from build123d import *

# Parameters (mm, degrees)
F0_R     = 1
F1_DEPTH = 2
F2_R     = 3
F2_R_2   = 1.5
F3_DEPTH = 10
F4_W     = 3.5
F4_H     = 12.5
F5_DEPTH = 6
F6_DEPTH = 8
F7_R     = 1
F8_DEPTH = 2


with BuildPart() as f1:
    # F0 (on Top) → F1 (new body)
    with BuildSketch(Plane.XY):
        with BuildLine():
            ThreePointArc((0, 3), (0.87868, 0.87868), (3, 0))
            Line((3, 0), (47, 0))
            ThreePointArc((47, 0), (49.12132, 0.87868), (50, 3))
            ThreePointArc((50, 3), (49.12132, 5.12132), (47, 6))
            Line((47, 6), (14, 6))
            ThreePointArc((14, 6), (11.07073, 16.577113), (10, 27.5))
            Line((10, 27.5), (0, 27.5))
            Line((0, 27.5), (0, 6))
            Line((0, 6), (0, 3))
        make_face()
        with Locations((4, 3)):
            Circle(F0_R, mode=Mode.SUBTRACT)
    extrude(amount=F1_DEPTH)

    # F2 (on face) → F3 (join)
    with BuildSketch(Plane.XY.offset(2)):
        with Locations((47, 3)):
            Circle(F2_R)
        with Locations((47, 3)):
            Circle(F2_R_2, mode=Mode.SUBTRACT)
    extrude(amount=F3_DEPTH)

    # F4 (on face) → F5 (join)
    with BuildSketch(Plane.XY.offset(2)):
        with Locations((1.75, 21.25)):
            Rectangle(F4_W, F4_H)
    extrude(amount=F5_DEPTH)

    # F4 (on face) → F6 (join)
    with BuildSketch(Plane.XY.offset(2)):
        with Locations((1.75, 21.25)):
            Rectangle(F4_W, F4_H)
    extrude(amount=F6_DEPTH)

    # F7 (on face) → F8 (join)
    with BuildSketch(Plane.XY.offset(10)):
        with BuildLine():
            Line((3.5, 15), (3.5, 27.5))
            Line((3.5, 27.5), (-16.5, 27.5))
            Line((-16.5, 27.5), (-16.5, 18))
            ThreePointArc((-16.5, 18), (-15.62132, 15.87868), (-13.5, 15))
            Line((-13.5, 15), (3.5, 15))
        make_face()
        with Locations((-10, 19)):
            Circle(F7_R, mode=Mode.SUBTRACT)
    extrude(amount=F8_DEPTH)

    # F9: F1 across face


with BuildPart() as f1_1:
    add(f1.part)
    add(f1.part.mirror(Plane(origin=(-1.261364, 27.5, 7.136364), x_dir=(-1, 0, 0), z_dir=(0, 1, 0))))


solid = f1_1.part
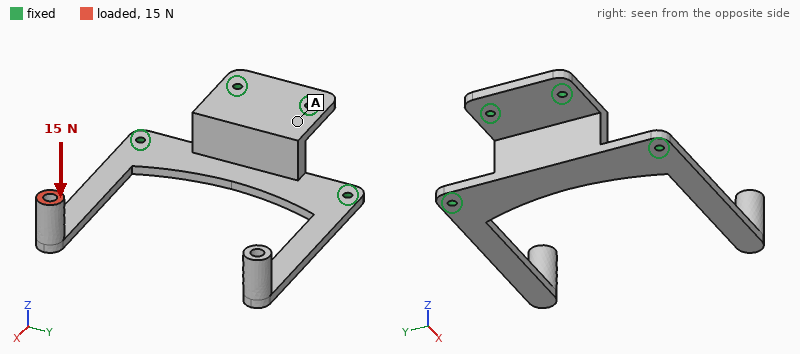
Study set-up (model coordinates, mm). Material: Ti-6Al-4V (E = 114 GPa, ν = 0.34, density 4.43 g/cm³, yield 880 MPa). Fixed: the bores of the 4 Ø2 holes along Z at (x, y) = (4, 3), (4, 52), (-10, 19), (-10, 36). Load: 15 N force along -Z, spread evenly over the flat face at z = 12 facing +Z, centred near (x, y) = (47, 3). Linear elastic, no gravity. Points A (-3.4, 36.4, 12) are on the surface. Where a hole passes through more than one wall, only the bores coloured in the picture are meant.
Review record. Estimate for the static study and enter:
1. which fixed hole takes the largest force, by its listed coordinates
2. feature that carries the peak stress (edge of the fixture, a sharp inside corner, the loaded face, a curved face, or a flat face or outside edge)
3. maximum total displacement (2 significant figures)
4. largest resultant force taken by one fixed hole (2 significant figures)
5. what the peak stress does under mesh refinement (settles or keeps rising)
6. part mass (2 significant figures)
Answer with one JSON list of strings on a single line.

["(4, 3)", "edge of the fixture", "0.80 mm", "23 N", "keeps rising", "19 g"]
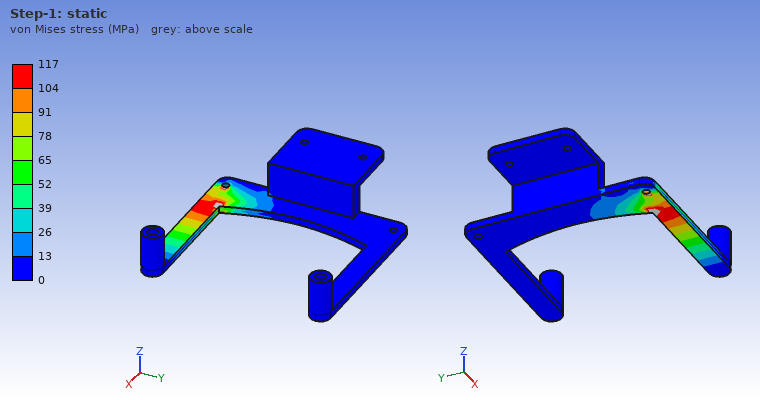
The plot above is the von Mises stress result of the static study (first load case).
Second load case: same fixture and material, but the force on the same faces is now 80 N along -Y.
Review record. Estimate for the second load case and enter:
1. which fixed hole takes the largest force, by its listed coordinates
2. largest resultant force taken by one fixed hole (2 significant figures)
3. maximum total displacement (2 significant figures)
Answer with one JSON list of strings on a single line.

["(4, 52)", "130 N", "1.0 mm"]
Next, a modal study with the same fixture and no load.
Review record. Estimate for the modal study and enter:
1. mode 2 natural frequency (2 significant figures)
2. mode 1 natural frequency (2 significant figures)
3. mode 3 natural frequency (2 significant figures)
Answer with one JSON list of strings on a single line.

["590 Hz", "580 Hz", "1700 Hz"]
